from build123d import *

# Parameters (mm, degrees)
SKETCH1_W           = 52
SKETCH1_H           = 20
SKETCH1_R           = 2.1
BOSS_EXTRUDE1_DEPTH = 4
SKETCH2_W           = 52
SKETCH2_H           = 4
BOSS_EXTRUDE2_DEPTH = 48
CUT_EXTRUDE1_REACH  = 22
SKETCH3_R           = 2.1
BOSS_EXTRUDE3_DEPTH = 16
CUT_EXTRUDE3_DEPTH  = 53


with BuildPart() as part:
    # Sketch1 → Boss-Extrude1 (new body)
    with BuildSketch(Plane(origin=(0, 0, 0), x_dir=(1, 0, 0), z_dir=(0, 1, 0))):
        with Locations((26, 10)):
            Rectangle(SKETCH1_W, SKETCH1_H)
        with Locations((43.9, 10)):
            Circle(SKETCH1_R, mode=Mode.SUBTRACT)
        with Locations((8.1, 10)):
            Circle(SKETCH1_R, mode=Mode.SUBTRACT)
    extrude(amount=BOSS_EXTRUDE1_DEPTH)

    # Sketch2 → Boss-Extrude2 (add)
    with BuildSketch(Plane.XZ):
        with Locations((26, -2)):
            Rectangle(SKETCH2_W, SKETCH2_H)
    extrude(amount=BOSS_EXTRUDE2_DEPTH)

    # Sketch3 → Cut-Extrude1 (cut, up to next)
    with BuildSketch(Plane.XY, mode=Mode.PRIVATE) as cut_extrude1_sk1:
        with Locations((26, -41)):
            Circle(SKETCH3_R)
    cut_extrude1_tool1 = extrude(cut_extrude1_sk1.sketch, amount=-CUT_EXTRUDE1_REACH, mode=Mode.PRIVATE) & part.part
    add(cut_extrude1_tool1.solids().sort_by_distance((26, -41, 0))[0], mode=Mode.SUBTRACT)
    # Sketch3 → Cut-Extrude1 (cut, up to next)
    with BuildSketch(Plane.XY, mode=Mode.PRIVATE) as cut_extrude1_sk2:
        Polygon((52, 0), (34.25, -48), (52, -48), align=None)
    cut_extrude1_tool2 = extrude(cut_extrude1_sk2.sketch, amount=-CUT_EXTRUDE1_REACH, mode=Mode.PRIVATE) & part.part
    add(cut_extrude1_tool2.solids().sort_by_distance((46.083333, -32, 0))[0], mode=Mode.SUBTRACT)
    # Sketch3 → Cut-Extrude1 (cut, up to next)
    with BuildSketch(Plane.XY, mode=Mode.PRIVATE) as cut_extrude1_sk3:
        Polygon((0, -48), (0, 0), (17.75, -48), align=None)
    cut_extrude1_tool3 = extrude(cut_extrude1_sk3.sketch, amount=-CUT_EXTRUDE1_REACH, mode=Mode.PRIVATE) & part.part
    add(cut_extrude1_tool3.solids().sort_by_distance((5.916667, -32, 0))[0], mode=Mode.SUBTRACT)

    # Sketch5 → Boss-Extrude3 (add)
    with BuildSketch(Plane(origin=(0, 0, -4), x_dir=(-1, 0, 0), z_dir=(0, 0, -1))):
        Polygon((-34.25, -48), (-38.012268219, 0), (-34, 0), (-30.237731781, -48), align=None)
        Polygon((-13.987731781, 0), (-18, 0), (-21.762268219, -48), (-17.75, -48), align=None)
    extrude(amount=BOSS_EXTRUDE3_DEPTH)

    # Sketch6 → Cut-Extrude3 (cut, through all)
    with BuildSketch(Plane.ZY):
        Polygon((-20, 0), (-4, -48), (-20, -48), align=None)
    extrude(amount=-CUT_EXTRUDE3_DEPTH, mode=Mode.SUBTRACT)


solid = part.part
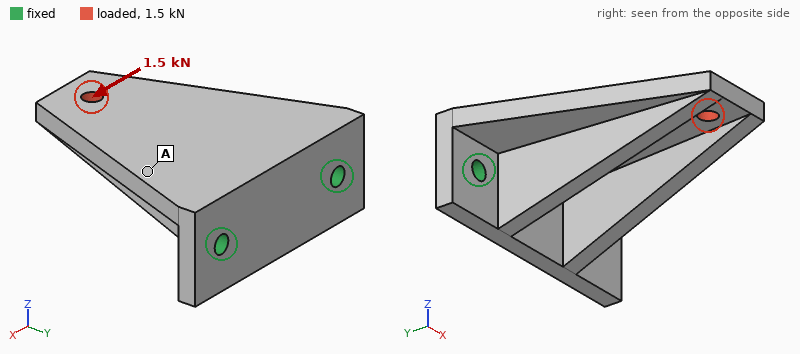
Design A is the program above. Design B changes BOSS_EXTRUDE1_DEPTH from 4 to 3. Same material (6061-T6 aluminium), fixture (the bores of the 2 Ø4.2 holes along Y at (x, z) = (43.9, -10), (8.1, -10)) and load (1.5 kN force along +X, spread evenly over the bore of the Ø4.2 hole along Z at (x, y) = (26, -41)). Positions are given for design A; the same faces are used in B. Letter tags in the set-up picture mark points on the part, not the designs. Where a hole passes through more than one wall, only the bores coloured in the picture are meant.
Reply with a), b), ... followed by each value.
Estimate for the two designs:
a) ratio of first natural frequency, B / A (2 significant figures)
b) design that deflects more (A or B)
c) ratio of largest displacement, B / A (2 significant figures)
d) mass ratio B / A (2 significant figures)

a) 0.77
b) B
c) 1.3
d) 0.93
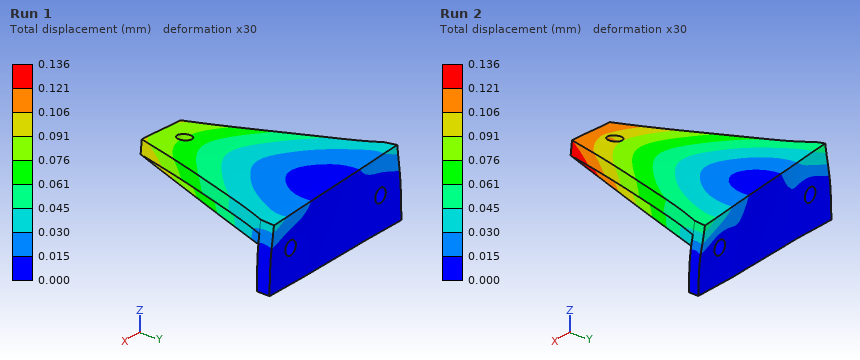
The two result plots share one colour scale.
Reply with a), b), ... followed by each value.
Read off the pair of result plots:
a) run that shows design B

a) Run 2
